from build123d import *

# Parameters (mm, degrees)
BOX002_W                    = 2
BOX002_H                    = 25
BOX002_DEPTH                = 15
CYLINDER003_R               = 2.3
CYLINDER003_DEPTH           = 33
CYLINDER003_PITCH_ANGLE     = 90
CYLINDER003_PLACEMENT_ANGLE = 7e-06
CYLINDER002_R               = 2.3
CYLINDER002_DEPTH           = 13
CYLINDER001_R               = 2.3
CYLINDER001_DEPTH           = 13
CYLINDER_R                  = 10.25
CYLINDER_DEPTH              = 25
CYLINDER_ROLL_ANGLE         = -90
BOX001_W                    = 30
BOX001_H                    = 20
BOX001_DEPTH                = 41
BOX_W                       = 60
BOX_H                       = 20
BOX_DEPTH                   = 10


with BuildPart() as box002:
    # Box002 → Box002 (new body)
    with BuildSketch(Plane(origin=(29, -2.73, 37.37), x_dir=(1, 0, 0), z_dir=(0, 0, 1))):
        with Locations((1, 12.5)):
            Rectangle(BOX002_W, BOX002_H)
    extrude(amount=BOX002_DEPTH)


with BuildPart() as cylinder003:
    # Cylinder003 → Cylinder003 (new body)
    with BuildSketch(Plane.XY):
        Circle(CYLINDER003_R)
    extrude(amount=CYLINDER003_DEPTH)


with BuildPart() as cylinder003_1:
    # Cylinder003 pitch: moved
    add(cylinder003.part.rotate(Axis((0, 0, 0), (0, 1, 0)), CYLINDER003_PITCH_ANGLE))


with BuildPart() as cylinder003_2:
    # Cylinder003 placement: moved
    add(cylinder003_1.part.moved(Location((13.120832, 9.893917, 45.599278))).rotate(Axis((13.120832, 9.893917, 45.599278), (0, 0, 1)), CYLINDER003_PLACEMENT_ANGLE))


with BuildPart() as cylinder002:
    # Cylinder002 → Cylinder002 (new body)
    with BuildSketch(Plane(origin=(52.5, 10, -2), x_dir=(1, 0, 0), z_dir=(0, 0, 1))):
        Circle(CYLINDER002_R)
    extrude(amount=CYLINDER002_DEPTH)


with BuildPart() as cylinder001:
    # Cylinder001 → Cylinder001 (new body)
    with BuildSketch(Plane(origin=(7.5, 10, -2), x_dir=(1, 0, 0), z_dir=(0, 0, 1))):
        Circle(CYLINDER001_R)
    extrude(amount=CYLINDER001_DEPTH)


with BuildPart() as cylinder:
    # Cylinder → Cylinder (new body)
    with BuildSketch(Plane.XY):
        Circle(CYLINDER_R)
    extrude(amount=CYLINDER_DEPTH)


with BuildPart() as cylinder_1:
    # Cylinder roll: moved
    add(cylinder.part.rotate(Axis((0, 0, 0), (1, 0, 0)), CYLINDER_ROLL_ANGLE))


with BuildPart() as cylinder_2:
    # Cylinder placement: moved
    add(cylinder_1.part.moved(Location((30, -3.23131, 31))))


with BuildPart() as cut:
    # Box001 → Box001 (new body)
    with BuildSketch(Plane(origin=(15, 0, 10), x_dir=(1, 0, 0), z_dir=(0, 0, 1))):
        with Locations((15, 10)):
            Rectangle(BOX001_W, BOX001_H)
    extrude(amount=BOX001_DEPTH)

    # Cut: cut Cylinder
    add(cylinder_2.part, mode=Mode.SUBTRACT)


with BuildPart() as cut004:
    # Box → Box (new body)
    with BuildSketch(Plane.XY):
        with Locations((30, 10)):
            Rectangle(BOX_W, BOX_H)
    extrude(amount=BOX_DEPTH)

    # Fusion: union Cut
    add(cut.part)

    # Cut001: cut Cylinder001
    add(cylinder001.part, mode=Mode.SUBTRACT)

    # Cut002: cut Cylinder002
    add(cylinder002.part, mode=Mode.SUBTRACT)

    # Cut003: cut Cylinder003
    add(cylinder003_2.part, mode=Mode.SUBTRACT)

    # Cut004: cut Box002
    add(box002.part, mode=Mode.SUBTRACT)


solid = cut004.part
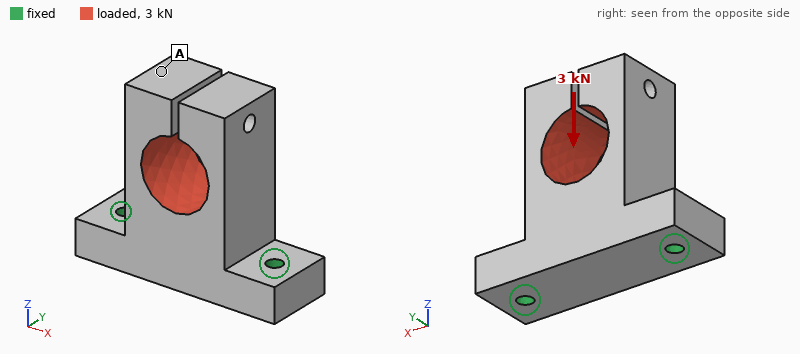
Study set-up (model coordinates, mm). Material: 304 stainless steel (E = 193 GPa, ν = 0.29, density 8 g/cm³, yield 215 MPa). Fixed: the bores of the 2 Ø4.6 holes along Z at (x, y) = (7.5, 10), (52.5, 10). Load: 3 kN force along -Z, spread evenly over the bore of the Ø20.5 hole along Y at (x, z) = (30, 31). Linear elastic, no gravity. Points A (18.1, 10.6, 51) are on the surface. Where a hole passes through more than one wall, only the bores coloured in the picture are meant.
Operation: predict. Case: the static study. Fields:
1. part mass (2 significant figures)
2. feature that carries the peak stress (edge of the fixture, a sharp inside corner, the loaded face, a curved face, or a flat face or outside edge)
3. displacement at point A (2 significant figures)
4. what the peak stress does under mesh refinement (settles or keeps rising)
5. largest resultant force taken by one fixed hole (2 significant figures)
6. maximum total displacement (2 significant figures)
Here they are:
230 g
edge of the fixture
28 µm
keeps rising
1.6 kN
33 µm
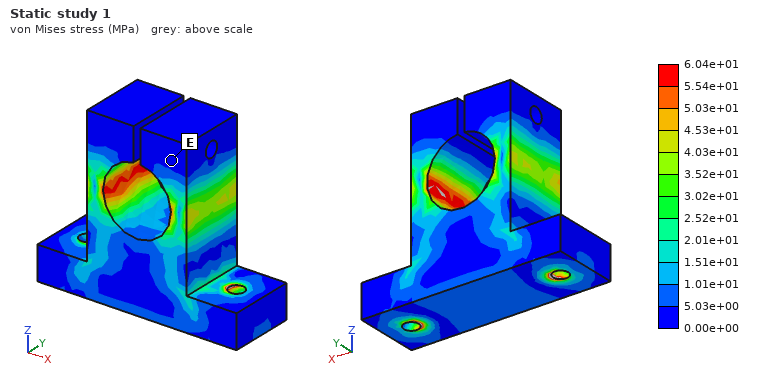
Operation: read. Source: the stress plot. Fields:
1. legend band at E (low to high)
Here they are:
0.00e+00 to 5.03e+00 MPa
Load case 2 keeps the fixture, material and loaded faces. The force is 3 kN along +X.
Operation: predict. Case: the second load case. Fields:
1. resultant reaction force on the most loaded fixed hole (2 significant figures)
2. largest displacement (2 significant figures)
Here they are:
2.5 kN
59 µm
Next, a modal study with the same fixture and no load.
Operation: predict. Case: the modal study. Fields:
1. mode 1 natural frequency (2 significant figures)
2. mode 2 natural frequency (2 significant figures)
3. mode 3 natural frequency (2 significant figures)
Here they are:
3100 Hz
3200 Hz
3300 Hz
